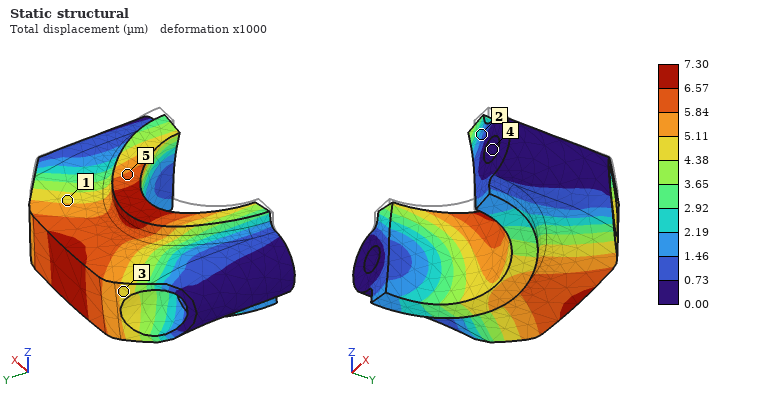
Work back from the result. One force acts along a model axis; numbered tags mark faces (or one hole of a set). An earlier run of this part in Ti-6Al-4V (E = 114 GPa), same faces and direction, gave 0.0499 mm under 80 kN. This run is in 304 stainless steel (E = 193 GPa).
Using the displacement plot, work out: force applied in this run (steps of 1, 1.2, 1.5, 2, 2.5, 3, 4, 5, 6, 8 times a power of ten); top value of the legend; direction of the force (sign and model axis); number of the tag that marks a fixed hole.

20 kN
7.30 µm
-Z
4
